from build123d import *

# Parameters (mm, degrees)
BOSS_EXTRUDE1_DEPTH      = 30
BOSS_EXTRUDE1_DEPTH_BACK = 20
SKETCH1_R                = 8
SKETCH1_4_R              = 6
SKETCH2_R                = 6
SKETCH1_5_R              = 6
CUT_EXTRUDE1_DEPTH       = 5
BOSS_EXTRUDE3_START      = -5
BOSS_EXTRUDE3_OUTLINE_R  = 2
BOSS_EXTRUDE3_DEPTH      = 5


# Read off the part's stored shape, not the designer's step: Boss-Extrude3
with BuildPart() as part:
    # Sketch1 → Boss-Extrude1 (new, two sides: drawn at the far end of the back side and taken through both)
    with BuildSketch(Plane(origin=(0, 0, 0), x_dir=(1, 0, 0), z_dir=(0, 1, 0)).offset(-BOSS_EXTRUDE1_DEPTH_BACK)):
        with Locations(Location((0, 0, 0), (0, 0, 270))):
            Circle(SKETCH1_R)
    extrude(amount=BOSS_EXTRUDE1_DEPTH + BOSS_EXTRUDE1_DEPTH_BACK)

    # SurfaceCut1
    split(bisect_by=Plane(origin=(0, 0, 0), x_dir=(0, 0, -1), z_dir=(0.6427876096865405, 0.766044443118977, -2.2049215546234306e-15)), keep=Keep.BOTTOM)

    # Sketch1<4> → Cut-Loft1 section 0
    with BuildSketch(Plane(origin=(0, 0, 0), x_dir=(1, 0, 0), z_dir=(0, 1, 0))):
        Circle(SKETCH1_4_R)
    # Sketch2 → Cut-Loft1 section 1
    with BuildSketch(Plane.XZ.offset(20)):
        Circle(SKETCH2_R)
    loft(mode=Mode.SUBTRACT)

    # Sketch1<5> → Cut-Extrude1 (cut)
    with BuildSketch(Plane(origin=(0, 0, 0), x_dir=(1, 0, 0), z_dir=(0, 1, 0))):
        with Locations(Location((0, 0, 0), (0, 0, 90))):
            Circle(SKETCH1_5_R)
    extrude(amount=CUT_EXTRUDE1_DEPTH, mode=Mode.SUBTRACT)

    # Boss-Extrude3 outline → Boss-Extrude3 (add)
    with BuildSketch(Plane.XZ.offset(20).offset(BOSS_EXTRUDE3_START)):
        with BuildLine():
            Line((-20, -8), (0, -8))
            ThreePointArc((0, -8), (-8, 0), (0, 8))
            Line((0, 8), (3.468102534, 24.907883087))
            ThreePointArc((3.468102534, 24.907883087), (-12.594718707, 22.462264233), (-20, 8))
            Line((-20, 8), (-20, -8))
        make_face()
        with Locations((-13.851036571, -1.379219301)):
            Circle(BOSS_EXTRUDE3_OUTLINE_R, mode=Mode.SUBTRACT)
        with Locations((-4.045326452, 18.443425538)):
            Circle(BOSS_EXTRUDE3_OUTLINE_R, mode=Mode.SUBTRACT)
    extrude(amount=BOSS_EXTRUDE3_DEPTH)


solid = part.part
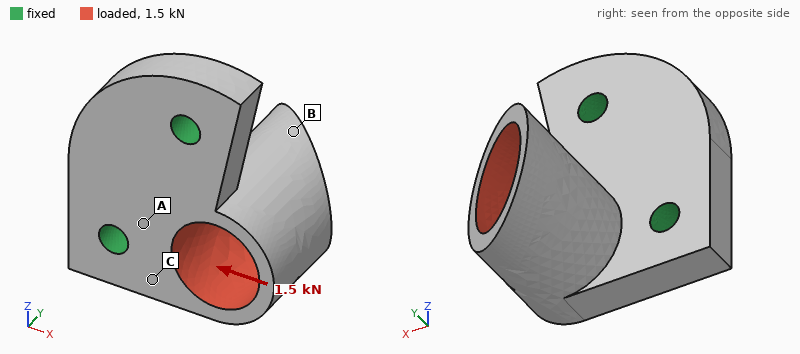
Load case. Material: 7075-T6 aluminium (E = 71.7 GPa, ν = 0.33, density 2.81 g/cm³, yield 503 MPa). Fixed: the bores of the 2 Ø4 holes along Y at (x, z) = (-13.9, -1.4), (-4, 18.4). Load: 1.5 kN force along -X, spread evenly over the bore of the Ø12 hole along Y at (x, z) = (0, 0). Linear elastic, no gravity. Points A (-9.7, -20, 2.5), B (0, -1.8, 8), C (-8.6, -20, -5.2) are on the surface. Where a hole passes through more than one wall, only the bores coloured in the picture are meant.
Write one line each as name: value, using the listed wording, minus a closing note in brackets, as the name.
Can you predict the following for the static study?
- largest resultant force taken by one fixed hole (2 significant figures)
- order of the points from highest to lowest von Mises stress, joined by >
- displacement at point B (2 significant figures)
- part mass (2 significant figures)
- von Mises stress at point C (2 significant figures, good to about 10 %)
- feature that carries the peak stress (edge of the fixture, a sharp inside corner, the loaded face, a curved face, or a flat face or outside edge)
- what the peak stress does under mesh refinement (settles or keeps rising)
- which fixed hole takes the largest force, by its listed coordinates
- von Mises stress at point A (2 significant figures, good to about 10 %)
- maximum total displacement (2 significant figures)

largest resultant force taken by one fixed hole: 1.3 kN
order of the points from highest to lowest von Mises stress, joined by >: C > A > B
displacement at point B: 0.13 mm
part mass: 12 g
von Mises stress at point C: 110 MPa
feature that carries the peak stress: edge of the fixture
what the peak stress does under mesh refinement: keeps rising
which fixed hole takes the largest force, by its listed coordinates: (-13.9, -1.4)
von Mises stress at point A: 51 MPa
maximum total displacement: 0.20 mm
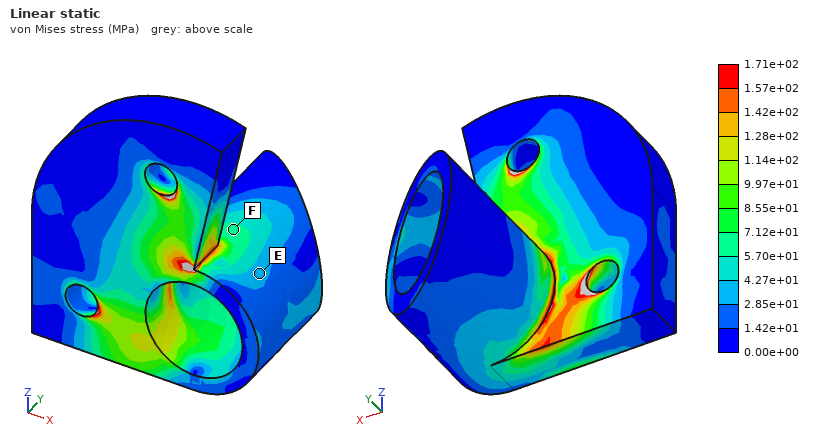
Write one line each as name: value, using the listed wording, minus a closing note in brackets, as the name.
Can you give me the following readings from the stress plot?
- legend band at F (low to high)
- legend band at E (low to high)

legend band at F: 5.70e+01 to 7.12e+01 MPa
legend band at E: 2.85e+01 to 4.27e+01 MPa
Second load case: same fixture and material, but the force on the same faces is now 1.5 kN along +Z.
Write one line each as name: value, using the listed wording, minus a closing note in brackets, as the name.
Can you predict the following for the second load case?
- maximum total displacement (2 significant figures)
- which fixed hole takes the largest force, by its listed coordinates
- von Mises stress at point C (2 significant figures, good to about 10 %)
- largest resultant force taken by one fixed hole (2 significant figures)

maximum total displacement: 0.11 mm
which fixed hole takes the largest force, by its listed coordinates: (-4, 18.4)
von Mises stress at point C: 79 MPa
largest resultant force taken by one fixed hole: 1.1 kN
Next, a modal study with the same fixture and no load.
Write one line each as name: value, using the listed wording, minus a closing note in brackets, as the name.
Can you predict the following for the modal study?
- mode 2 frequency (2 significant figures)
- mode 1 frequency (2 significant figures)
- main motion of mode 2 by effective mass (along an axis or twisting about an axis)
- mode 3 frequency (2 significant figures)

mode 2 frequency: 11 kHz
mode 1 frequency: 6400 Hz
main motion of mode 2 by effective mass: along Z
mode 3 frequency: 16 kHz
